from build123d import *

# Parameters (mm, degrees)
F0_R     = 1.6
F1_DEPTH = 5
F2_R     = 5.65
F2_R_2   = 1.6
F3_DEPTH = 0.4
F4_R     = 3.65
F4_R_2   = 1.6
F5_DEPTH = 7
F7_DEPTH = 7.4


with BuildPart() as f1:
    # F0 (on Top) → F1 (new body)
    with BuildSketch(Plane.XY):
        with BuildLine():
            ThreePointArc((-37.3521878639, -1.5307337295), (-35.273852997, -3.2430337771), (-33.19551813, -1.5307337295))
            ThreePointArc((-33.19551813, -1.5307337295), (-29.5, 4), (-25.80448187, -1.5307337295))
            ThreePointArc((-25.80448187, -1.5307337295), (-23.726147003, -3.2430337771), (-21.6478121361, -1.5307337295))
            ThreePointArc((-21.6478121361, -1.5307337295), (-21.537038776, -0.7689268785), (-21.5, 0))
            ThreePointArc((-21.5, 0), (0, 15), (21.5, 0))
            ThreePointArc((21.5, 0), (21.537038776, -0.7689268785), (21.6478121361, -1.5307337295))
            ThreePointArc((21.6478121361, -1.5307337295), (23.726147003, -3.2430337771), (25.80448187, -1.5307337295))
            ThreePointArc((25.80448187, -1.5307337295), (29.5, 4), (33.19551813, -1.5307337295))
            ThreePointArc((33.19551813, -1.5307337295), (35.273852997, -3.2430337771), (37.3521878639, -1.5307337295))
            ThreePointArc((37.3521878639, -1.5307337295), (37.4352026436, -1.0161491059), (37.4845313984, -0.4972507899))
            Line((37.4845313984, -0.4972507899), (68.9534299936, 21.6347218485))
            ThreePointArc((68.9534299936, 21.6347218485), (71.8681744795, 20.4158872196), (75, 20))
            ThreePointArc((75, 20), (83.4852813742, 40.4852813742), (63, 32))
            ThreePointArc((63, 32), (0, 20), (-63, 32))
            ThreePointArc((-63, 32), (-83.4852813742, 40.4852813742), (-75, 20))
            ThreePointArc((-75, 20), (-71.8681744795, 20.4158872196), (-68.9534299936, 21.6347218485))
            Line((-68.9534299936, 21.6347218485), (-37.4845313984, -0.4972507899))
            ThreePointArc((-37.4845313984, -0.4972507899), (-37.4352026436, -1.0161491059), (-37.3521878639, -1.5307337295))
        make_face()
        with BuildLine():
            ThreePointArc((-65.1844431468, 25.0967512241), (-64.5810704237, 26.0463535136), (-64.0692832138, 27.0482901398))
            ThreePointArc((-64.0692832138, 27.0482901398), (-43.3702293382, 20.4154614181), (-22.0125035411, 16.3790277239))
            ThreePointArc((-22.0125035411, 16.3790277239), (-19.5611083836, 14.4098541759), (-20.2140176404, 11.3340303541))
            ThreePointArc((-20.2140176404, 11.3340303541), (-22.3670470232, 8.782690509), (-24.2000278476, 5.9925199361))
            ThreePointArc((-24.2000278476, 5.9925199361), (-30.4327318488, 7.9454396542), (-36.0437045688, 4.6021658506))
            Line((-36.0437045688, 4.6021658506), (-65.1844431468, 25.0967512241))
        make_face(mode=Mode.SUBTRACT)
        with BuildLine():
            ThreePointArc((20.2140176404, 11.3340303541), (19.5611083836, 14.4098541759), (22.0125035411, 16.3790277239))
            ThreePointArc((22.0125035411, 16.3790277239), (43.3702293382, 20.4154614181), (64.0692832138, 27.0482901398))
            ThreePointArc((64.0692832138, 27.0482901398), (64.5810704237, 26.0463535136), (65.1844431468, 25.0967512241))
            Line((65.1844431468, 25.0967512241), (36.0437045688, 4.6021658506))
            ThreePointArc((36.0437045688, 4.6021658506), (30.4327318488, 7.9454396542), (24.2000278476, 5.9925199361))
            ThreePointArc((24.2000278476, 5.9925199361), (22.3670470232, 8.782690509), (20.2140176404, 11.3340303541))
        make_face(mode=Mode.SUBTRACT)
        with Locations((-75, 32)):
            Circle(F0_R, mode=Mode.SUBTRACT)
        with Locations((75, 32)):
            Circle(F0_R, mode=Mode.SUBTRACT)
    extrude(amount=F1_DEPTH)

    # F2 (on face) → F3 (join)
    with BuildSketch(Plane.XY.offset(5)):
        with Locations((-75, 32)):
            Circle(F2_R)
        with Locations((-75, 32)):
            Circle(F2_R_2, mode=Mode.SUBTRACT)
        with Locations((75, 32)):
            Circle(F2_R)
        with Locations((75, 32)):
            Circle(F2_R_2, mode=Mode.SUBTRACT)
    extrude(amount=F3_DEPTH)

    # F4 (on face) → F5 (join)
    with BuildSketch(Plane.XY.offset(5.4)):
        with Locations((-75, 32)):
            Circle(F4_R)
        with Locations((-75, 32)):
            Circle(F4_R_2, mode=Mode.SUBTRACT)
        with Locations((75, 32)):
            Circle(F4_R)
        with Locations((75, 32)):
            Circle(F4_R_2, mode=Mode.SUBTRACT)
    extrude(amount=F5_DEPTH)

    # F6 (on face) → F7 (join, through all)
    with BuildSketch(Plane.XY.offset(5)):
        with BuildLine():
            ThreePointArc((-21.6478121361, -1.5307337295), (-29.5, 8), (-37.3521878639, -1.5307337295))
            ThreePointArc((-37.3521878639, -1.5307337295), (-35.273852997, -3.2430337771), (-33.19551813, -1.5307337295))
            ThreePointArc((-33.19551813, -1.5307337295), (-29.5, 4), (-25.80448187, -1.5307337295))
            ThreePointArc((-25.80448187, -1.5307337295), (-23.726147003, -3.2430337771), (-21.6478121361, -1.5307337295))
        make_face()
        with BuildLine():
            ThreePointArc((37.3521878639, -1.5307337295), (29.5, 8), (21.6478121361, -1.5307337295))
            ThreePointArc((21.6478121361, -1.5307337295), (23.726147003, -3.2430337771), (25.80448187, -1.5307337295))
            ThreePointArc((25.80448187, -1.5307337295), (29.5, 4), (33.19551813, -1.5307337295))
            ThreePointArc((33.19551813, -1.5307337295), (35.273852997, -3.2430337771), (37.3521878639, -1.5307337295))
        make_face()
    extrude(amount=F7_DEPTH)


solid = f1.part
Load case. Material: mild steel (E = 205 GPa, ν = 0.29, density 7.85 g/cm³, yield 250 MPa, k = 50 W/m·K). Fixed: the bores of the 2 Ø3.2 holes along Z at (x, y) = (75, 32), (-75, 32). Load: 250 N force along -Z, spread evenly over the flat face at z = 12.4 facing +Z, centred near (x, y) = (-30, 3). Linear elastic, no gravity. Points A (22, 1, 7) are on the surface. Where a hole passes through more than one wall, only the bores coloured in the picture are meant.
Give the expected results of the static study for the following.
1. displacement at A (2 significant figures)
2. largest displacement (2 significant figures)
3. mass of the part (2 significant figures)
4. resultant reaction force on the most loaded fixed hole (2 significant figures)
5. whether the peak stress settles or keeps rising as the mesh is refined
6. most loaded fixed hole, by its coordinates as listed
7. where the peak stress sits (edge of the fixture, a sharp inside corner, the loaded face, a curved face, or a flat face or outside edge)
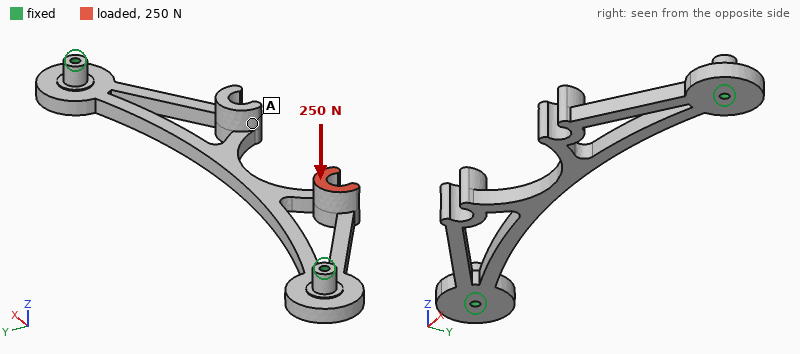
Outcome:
0.16 mm
0.31 mm
110 g
200 N
keeps rising
(-75, 32)
edge of the fixture
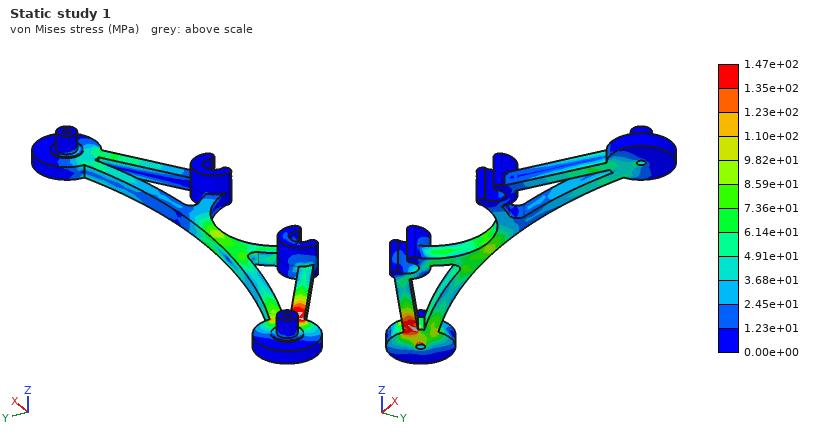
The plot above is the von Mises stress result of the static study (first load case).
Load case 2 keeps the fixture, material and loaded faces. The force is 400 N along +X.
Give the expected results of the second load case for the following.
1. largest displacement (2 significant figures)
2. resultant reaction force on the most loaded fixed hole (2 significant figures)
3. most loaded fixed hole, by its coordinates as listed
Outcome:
79 µm
320 N
(75, 32)
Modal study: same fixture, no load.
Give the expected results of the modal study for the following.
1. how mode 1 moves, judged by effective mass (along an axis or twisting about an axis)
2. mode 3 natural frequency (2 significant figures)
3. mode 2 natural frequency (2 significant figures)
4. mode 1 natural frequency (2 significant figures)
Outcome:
along Z
2300 Hz
1900 Hz
920 Hz
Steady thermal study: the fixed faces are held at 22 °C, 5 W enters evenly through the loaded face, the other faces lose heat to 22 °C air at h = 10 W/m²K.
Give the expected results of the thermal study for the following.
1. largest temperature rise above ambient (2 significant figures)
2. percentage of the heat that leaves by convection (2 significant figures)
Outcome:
75 K
34 %
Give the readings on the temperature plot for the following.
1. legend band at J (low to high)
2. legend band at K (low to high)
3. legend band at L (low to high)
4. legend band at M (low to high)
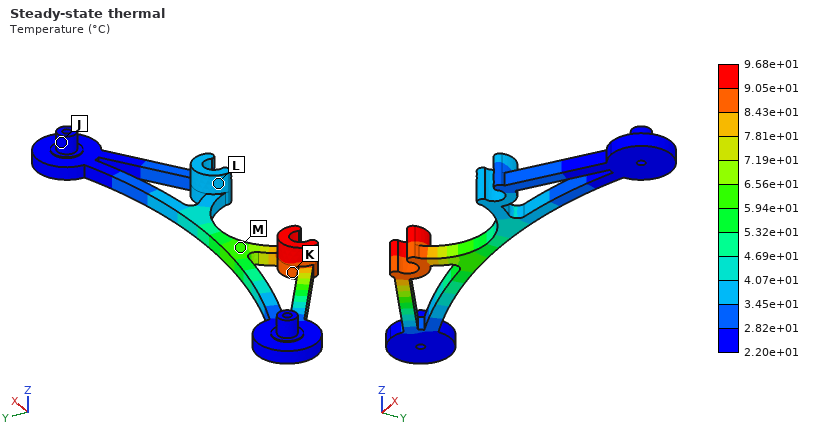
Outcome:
2.20e+01 to 2.82e+01 °C
8.43e+01 to 9.05e+01 °C
3.45e+01 to 4.07e+01 °C
5.94e+01 to 6.56e+01 °C
